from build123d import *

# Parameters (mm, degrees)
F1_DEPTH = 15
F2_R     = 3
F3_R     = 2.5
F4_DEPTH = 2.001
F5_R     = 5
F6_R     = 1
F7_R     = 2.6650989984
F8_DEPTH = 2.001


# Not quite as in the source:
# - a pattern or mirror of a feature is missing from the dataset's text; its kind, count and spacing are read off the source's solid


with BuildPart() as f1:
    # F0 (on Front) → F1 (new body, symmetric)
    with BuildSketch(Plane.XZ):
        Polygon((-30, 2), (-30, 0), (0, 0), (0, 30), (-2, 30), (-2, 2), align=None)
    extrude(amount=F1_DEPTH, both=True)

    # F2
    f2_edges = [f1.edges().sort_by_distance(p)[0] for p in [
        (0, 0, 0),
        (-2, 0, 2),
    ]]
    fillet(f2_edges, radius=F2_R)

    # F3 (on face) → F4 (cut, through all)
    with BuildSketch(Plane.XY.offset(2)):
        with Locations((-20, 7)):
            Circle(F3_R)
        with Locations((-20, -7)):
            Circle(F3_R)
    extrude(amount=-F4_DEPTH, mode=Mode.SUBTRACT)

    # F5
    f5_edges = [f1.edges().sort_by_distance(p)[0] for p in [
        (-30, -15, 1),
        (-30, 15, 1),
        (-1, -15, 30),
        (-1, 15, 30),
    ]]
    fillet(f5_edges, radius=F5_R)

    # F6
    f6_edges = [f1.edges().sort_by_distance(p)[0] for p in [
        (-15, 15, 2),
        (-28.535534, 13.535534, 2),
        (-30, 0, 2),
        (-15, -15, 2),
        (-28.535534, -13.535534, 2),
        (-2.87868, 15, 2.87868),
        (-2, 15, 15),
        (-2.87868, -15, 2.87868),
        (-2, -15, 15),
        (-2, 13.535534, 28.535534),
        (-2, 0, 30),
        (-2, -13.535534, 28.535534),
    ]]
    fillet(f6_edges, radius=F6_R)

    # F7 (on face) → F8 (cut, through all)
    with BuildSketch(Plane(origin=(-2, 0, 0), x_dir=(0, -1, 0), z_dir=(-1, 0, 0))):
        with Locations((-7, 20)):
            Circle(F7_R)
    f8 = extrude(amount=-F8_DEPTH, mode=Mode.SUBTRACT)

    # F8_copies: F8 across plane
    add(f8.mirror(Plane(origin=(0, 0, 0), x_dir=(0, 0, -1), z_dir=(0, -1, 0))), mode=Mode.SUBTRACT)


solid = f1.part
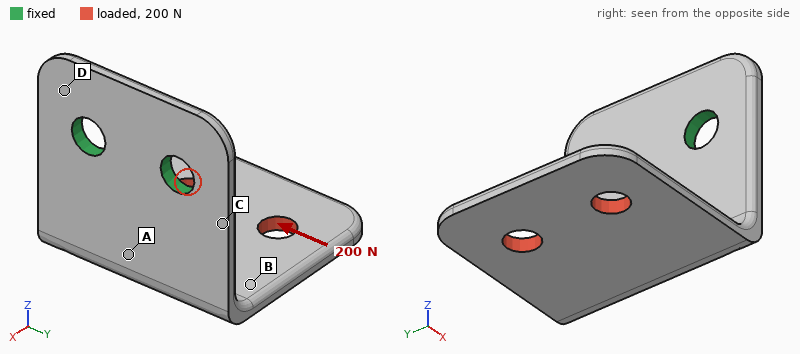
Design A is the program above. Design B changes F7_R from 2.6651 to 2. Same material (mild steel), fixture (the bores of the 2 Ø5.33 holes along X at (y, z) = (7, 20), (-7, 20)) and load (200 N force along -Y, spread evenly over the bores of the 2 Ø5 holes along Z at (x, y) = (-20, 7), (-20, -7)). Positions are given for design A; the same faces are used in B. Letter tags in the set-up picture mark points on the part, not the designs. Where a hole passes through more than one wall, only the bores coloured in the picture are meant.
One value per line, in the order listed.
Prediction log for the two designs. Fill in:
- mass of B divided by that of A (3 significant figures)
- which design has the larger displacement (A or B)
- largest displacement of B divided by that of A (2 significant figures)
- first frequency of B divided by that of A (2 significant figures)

1.01
B
1.1
0.97
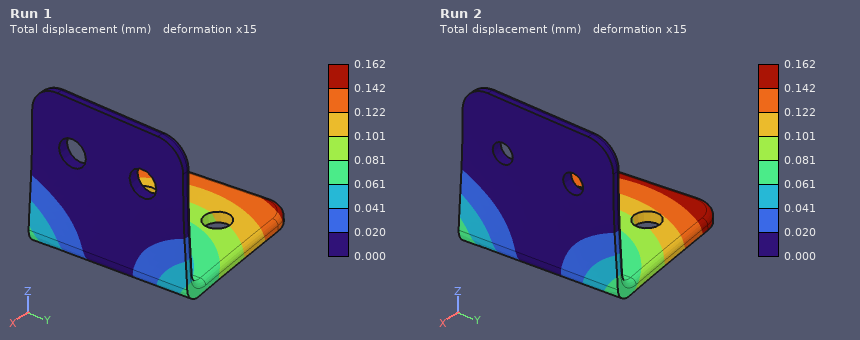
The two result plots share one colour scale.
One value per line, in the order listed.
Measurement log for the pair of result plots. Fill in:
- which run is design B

Run 2
